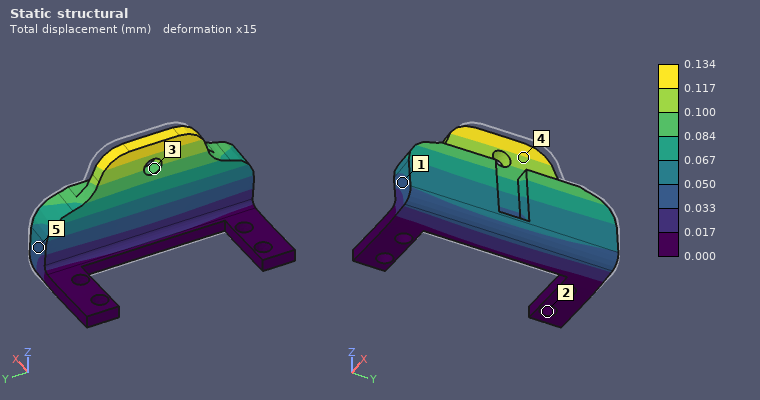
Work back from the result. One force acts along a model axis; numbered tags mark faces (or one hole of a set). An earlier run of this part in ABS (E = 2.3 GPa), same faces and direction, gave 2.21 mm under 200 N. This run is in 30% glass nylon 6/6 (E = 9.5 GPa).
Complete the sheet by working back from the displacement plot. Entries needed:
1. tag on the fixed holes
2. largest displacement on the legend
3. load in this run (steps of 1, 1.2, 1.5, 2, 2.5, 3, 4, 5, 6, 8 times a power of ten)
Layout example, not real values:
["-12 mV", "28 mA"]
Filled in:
["2", "0.134 mm", "50 N"]
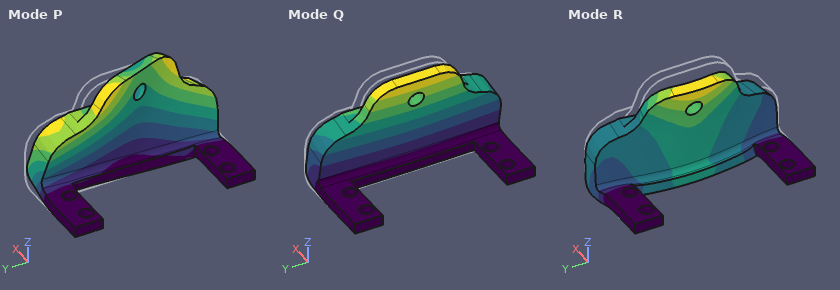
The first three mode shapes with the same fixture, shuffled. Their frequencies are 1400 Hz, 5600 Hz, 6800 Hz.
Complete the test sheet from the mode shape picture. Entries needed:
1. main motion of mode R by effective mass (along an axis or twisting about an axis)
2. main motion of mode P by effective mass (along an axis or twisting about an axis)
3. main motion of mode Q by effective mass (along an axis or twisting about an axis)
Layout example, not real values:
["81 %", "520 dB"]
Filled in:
["along Z", "along Y", "along X"]
